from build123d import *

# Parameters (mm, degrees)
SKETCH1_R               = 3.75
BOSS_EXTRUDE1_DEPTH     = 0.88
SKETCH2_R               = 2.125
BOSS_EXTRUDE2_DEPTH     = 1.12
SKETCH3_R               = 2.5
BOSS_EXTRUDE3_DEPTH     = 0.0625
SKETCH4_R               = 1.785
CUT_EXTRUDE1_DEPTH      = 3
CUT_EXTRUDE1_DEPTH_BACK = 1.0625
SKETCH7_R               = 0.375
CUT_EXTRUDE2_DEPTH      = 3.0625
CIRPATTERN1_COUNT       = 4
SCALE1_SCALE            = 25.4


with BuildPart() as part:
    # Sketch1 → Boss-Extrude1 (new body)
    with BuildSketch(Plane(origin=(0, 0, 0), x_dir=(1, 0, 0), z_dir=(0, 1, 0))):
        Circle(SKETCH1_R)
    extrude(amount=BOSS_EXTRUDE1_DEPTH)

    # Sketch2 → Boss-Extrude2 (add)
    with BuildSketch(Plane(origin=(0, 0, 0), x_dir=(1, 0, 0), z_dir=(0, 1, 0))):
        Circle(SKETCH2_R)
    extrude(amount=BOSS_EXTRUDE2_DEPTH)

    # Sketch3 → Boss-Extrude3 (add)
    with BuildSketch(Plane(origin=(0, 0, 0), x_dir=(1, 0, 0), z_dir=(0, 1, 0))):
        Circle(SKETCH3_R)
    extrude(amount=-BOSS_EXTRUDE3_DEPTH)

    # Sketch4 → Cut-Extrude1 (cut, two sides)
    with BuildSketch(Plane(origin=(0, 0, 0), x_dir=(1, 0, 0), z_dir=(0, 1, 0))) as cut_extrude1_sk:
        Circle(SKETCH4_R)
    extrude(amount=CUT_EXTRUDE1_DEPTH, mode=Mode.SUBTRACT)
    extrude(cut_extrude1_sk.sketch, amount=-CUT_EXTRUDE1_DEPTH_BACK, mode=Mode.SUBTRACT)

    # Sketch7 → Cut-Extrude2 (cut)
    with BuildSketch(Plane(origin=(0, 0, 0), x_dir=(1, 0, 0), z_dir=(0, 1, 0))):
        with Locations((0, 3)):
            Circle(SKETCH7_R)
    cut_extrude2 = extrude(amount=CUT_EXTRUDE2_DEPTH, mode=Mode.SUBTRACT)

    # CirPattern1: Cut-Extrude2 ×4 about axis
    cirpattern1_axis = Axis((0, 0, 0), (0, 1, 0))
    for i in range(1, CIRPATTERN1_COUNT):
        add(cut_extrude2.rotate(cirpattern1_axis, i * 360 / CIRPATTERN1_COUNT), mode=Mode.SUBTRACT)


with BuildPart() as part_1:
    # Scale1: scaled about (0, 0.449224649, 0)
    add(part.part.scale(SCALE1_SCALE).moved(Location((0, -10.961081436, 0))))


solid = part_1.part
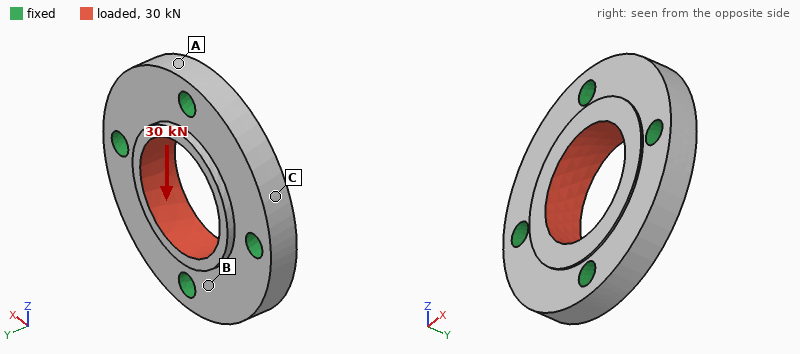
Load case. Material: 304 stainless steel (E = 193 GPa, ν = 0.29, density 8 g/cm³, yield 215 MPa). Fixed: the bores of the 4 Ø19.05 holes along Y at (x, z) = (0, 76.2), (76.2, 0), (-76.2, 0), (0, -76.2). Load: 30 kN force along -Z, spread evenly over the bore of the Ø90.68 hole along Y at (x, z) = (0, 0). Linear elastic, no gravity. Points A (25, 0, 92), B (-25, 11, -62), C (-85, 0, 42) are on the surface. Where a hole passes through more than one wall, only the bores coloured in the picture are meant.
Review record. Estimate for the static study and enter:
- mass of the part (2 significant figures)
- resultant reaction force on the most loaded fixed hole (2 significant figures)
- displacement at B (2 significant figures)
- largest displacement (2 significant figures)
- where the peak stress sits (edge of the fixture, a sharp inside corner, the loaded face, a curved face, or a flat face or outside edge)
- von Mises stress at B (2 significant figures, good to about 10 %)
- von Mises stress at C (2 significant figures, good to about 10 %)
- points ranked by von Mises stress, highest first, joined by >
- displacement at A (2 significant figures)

3.9 kg
7.6 kN
1.2 µm
2.6 µm
edge of the fixture
5.7 MPa
3.0 MPa
B > C > A
0.71 µm
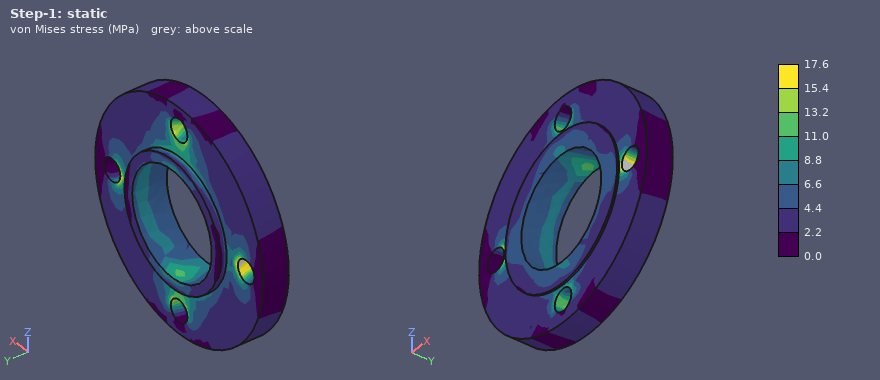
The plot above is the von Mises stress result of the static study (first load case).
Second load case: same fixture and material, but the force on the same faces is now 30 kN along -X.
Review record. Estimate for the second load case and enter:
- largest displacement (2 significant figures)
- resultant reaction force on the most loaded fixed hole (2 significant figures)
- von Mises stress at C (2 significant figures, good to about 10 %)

2.6 µm
7.6 kN
2.8 MPa
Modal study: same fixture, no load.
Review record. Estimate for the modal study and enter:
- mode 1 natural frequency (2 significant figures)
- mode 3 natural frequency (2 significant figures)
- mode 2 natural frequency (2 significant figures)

6900 Hz
7200 Hz
7200 Hz
